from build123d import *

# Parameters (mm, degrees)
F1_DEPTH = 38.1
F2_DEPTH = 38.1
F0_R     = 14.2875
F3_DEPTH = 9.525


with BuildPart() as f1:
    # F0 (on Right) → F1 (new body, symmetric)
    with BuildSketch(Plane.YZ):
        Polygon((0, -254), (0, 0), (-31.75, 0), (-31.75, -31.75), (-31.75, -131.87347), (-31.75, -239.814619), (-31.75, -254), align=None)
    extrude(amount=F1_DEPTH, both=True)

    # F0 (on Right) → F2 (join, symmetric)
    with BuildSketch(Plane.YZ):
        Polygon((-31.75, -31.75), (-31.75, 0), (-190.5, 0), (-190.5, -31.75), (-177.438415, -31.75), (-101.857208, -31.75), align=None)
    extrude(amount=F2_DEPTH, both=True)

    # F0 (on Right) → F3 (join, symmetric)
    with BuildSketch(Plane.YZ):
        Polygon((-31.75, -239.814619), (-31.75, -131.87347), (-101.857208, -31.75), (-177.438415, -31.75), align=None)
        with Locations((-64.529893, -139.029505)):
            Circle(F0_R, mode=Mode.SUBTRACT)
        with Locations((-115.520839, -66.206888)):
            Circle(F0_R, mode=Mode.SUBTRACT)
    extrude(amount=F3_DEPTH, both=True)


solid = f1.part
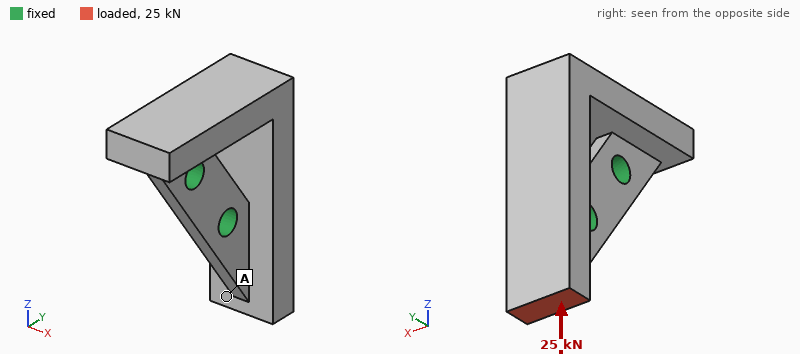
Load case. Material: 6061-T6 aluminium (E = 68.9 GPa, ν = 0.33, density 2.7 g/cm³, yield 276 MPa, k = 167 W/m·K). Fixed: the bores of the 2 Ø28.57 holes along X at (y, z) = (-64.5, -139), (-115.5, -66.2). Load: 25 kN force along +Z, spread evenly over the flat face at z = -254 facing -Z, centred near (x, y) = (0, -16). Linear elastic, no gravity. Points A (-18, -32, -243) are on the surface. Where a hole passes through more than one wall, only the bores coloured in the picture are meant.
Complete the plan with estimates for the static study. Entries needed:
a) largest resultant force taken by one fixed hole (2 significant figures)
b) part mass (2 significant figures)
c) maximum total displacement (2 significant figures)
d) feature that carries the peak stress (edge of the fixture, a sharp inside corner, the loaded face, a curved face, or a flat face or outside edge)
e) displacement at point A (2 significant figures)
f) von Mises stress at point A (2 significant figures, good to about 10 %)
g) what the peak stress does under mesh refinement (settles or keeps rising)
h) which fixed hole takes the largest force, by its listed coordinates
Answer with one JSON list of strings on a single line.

["24 kN", "3.2 kg", "0.14 mm", "edge of the fixture", "0.11 mm", "9.9 MPa", "keeps rising", "(-64.5, -139)"]
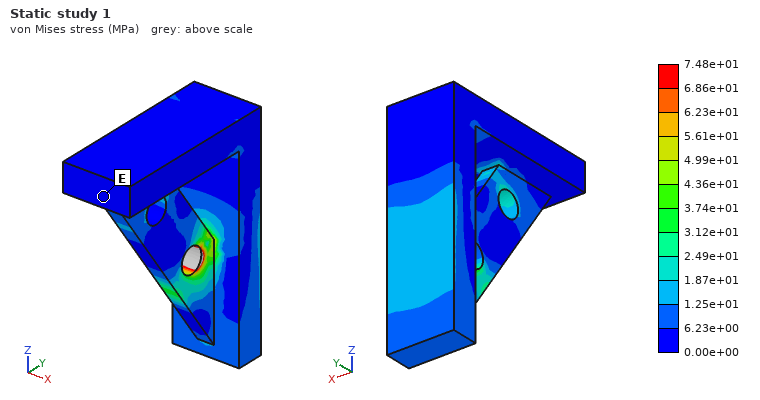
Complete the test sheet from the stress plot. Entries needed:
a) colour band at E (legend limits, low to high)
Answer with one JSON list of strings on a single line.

["0.00e+00 to 6.23e+00 MPa"]
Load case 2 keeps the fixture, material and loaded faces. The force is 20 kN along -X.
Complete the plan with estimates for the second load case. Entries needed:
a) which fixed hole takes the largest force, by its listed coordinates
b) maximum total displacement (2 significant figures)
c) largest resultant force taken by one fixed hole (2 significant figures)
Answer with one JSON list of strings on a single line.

["(-64.5, -139)", "0.87 mm", "31 kN"]
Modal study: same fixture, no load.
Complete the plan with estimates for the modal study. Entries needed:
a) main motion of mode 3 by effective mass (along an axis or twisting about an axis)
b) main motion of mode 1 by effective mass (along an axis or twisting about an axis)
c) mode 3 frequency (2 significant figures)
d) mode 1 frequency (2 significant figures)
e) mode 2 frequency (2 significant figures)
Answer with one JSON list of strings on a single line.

["along Z", "along X", "1800 Hz", "840 Hz", "1400 Hz"]
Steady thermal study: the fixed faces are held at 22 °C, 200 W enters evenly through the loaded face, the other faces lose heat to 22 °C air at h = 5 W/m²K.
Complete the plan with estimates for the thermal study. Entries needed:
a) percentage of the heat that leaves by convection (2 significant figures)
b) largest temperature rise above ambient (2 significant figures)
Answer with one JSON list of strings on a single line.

["4.6 %", "64 K"]
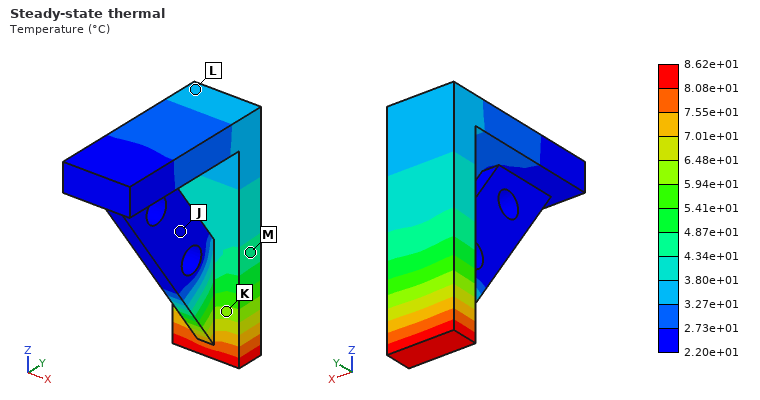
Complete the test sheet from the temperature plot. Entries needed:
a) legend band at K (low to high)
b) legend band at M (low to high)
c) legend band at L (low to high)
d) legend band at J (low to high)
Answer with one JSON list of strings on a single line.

["5.94e+01 to 6.48e+01 °C", "4.34e+01 to 4.87e+01 °C", "3.27e+01 to 3.80e+01 °C", "2.20e+01 to 2.73e+01 °C"]
